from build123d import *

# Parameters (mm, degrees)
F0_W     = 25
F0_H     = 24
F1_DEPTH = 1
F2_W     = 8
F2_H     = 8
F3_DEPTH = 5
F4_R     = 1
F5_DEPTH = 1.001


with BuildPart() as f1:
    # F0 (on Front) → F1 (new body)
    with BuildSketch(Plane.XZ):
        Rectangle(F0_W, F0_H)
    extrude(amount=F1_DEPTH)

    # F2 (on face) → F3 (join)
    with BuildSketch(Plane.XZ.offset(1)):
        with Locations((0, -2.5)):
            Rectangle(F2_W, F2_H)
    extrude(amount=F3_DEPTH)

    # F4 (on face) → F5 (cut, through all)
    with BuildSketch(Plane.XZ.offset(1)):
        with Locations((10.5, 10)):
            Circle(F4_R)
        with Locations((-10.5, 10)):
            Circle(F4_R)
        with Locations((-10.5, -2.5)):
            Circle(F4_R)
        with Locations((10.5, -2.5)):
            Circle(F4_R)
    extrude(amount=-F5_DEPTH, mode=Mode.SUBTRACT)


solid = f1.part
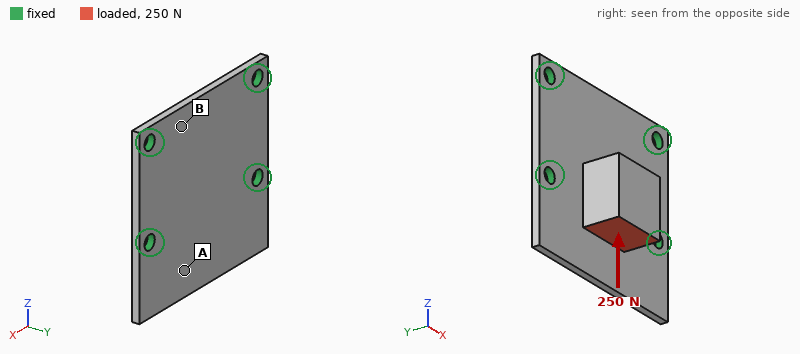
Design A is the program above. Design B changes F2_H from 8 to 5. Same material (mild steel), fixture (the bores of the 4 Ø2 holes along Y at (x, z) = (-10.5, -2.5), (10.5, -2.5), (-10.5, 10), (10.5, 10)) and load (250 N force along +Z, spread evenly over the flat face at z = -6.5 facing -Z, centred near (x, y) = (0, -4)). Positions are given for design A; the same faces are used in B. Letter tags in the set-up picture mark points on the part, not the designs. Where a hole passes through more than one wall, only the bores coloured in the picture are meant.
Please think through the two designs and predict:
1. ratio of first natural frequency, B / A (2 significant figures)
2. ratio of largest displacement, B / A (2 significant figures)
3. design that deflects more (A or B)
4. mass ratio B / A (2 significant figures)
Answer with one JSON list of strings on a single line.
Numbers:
["1.0", "1.2", "B", "0.87"]
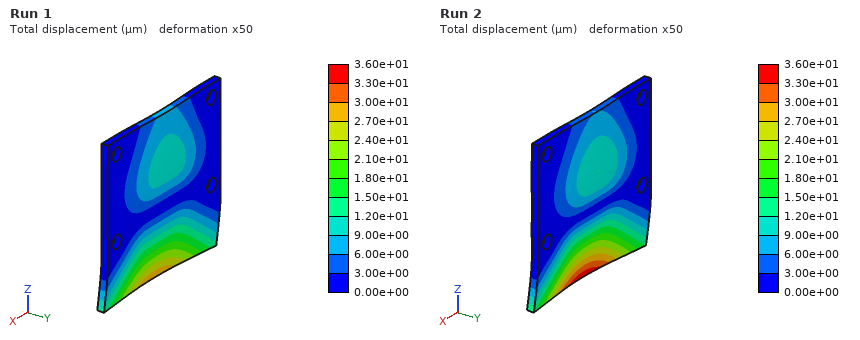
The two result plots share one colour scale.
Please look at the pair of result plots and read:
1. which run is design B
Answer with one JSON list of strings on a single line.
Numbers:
["Run 2"]
